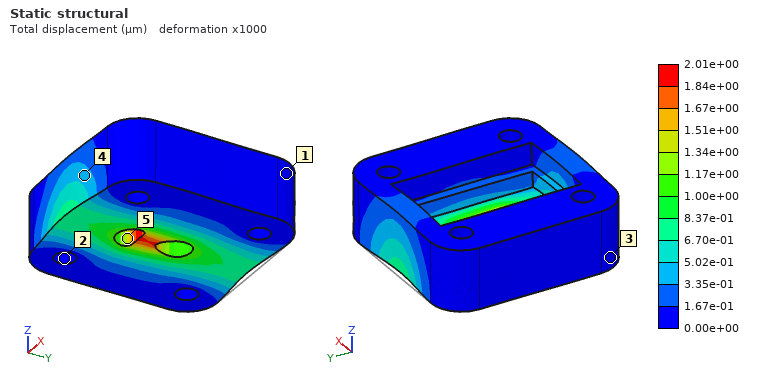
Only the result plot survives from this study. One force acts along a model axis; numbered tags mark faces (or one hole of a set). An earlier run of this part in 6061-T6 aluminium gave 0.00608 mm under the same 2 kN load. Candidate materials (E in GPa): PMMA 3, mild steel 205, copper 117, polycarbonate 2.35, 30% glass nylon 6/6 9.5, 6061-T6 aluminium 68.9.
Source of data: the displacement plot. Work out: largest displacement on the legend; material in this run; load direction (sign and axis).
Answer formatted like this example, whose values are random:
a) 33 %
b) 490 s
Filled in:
a) 2.01e+00 µm
b) mild steel
c) -Y
